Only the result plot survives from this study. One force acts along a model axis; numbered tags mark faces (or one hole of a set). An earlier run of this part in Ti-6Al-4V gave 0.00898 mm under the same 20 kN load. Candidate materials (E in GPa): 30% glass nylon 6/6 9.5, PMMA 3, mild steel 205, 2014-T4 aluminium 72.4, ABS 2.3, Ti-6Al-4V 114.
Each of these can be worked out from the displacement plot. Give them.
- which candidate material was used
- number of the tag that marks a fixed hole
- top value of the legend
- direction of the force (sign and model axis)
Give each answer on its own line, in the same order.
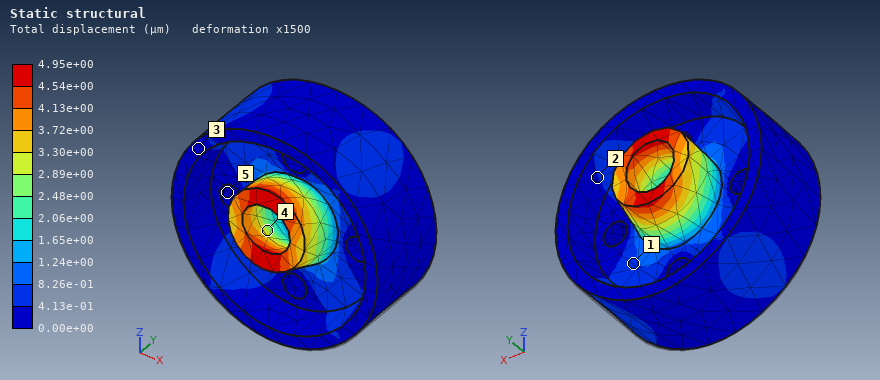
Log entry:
mild steel
5
4.95e+00 µm
+Z
